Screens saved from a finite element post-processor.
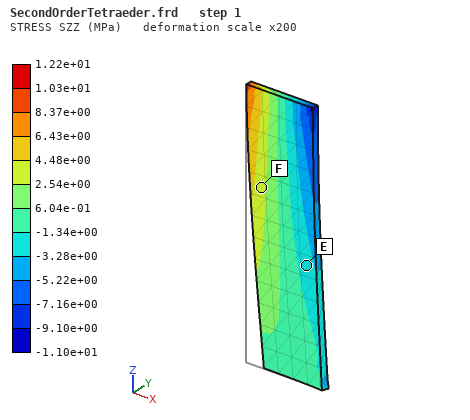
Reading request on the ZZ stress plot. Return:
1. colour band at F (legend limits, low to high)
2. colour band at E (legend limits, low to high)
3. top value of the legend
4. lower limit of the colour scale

2.54e+00 to 4.48e+00 MPa
-3.28e+00 to -1.34e+00 MPa
1.22e+01 MPa
-1.10e+01 MPa
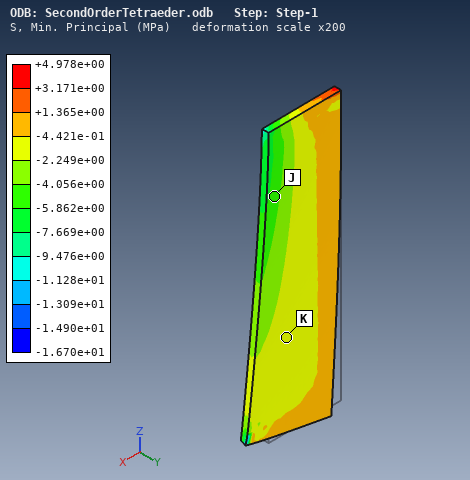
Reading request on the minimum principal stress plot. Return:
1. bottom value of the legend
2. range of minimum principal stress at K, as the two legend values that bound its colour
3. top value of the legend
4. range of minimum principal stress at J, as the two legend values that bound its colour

-1.670e+01 MPa
-2.249e+00 to -4.421e-01 MPa
+4.978e+00 MPa
-5.862e+00 to -4.056e+00 MPa
